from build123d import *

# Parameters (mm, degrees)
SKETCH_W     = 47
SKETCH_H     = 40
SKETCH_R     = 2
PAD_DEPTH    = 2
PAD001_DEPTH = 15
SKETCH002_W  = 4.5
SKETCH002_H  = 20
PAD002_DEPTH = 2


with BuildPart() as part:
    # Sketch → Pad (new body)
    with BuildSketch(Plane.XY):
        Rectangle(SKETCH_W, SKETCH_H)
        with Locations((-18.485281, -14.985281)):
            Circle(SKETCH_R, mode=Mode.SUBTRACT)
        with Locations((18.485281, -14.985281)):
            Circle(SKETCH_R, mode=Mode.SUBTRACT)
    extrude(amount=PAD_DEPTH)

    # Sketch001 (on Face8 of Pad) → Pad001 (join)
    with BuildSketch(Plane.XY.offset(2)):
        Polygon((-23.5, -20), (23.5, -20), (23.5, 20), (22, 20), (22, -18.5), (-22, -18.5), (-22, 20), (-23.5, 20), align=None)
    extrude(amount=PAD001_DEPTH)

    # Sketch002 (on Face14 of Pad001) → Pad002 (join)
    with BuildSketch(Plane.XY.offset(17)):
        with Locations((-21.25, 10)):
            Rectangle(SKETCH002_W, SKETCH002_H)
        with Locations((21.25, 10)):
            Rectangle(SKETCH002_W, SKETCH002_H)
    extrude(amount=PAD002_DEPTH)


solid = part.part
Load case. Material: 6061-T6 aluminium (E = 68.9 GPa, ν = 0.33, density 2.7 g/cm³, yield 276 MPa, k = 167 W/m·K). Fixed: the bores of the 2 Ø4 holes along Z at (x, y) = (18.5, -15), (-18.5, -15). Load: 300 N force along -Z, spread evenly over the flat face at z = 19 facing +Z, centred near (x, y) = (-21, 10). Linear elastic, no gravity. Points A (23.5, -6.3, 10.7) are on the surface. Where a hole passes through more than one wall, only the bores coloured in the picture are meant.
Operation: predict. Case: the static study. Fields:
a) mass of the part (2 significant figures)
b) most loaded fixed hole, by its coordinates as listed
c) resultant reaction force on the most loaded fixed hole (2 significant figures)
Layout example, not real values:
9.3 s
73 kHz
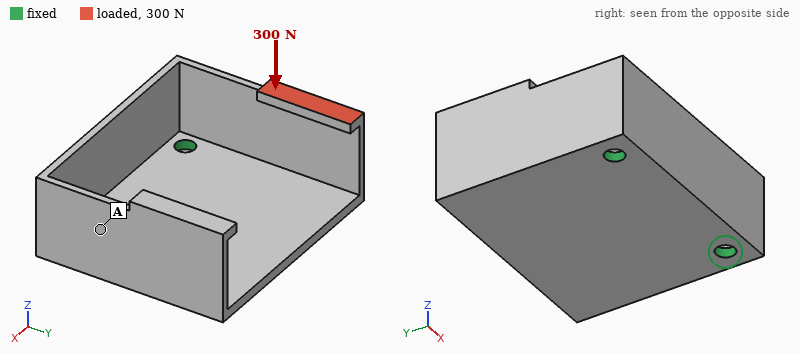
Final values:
19 g
(-18.5, -15)
280 N
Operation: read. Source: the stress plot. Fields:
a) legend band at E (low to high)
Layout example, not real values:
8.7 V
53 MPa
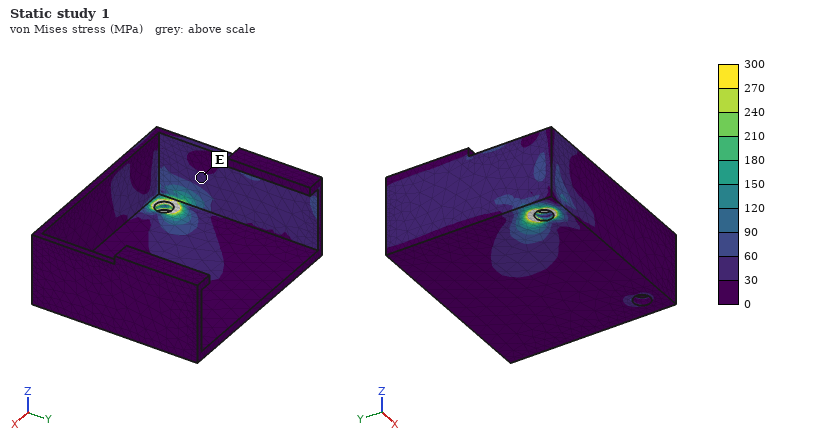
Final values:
30 to 60 MPa
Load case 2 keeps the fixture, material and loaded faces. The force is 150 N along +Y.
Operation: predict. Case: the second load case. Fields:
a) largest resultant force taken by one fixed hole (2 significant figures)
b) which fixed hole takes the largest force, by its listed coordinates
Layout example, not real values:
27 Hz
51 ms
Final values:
150 N
(-18.5, -15)
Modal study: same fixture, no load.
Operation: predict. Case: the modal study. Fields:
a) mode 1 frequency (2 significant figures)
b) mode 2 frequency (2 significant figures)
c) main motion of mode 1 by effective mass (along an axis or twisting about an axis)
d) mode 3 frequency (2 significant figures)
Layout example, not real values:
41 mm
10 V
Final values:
2000 Hz
2400 Hz
along Z
2600 Hz
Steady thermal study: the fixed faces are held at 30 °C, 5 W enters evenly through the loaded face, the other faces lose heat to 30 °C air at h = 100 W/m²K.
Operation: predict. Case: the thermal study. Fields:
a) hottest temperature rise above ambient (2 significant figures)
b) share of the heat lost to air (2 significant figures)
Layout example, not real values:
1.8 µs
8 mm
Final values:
18 K
43 %
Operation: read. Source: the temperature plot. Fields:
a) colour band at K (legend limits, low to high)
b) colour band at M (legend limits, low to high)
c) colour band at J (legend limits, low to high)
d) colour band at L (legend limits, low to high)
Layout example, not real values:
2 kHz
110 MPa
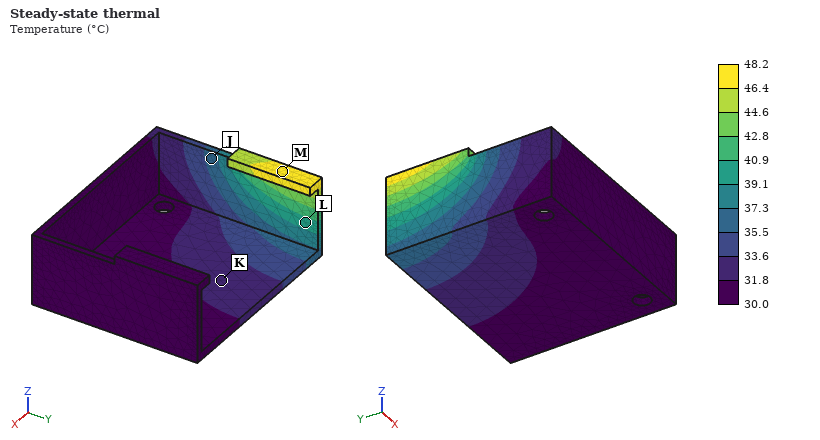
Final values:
31.8 to 33.6 °C
46.4 to 48.2 °C
35.5 to 37.3 °C
39.1 to 40.9 °C
